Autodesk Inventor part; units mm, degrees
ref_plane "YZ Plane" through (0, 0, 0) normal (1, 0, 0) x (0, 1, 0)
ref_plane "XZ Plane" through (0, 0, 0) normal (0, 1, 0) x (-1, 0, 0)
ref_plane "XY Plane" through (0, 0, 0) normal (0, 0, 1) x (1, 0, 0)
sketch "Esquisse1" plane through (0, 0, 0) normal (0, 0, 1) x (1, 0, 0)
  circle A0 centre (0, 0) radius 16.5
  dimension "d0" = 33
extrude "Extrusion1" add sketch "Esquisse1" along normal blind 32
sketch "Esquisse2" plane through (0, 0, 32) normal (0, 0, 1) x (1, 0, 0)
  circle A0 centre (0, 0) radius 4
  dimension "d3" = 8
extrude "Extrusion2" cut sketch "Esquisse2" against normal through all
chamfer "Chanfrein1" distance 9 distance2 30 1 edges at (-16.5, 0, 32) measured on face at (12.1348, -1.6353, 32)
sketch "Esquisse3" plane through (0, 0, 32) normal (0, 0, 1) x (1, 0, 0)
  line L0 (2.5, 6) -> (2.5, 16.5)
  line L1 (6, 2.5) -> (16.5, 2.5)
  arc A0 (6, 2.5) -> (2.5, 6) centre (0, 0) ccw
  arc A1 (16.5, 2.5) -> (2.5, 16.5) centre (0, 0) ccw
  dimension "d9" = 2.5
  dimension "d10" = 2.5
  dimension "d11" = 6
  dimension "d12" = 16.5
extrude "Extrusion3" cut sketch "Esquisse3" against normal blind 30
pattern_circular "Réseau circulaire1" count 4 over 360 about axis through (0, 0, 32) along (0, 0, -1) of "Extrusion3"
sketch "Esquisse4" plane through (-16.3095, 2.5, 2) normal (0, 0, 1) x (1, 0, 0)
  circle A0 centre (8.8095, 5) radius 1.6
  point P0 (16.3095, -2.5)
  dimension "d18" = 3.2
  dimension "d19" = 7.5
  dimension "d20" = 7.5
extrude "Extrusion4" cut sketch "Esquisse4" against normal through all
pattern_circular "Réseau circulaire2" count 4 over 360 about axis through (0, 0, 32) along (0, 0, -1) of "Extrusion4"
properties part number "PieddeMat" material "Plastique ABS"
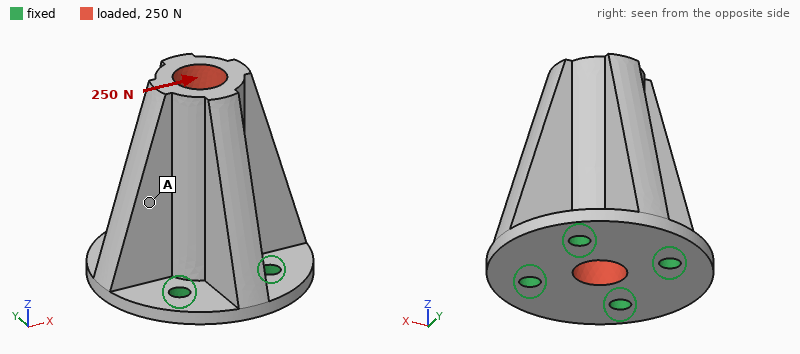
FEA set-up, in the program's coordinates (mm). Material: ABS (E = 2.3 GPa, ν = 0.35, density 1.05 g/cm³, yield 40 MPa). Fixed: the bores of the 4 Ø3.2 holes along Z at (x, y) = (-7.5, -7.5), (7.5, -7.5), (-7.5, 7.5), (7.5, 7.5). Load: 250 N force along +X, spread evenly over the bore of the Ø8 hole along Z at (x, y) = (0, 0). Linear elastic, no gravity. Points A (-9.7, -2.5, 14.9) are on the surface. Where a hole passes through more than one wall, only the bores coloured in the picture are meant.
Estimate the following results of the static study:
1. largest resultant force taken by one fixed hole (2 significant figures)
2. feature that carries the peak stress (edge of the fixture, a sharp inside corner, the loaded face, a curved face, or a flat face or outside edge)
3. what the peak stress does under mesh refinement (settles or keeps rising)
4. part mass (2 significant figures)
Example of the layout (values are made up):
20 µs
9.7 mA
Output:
140 N
edge of the fixture
keeps rising
7.7 g
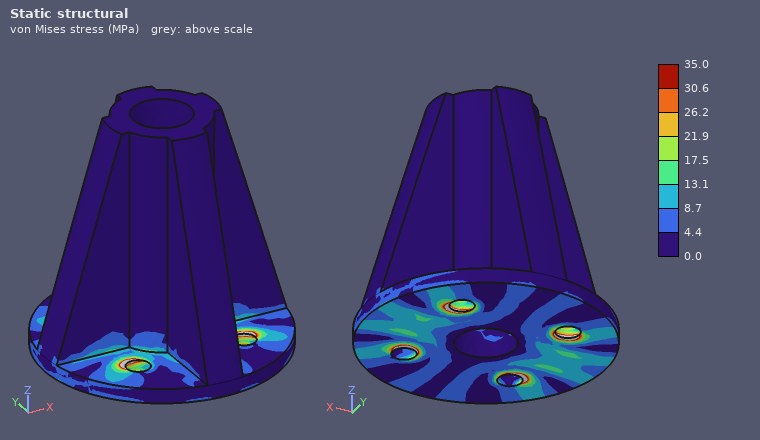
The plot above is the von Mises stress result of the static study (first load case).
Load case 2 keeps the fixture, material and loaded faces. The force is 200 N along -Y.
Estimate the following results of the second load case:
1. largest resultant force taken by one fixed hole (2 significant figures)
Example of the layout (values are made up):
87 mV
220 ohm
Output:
110 N
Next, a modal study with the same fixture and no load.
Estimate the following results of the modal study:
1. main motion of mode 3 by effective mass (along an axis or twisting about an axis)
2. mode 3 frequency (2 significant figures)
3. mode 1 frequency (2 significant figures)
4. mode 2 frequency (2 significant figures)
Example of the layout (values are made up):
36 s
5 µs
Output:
along Z
5200 Hz
2100 Hz
2100 Hz
